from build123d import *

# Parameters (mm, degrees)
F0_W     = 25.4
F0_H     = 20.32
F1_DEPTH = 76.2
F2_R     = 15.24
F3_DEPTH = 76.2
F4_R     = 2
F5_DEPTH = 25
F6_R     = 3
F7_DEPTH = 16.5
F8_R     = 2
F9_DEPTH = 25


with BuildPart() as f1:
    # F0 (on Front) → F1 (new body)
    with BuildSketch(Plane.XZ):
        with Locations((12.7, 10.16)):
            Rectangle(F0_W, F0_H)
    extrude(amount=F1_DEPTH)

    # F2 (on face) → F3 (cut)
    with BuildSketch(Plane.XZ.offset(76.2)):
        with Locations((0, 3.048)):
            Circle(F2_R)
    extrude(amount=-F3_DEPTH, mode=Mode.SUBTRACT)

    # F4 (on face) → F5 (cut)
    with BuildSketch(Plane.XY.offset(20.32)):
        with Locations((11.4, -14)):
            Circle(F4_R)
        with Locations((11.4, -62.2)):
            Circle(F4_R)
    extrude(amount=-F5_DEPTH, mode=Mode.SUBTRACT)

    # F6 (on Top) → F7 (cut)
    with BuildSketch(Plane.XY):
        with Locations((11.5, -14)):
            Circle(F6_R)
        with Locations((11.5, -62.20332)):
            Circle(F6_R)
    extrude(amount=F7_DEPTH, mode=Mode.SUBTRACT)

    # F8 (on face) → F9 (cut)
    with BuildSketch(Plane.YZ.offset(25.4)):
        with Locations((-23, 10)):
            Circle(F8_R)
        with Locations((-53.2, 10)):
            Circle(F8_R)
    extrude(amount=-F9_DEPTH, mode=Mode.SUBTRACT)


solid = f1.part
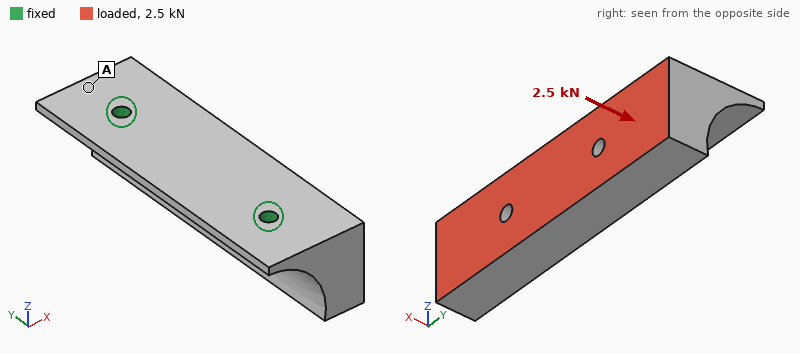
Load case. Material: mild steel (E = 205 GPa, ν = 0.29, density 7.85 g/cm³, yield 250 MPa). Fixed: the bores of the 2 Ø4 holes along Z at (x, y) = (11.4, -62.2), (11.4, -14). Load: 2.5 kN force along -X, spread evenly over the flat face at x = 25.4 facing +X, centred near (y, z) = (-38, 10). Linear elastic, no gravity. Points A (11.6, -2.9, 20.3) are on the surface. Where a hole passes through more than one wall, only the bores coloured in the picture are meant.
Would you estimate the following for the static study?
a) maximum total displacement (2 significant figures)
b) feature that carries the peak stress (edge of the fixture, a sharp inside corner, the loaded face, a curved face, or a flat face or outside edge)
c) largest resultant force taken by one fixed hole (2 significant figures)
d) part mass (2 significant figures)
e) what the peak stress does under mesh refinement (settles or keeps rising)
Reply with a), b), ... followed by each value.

a) 28 µm
b) edge of the fixture
c) 1.3 kN
d) 170 g
e) keeps rising
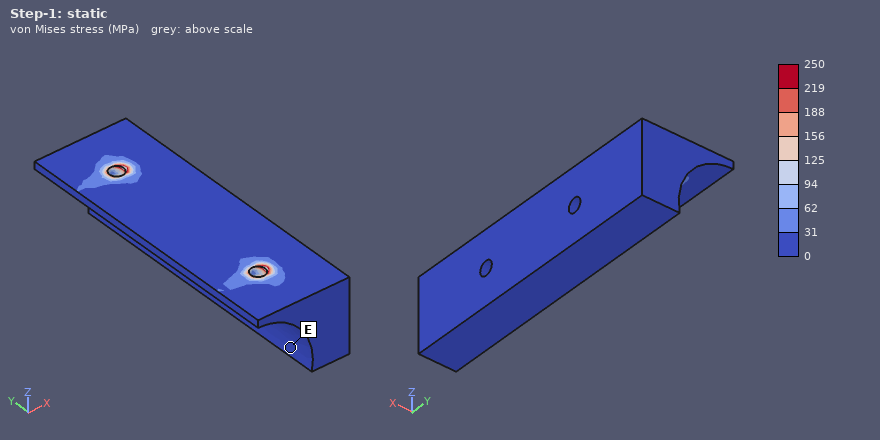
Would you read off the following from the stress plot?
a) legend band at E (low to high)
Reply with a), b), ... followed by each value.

a) 0 to 31 MPa
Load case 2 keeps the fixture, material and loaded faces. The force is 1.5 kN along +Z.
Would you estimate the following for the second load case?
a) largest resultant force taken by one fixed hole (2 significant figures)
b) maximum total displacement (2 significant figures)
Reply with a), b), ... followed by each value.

a) 750 N
b) 27 µm
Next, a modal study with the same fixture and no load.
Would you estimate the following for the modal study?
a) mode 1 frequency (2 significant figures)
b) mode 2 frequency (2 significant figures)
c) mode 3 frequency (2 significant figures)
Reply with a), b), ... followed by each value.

a) 4400 Hz
b) 9300 Hz
c) 13 kHz
